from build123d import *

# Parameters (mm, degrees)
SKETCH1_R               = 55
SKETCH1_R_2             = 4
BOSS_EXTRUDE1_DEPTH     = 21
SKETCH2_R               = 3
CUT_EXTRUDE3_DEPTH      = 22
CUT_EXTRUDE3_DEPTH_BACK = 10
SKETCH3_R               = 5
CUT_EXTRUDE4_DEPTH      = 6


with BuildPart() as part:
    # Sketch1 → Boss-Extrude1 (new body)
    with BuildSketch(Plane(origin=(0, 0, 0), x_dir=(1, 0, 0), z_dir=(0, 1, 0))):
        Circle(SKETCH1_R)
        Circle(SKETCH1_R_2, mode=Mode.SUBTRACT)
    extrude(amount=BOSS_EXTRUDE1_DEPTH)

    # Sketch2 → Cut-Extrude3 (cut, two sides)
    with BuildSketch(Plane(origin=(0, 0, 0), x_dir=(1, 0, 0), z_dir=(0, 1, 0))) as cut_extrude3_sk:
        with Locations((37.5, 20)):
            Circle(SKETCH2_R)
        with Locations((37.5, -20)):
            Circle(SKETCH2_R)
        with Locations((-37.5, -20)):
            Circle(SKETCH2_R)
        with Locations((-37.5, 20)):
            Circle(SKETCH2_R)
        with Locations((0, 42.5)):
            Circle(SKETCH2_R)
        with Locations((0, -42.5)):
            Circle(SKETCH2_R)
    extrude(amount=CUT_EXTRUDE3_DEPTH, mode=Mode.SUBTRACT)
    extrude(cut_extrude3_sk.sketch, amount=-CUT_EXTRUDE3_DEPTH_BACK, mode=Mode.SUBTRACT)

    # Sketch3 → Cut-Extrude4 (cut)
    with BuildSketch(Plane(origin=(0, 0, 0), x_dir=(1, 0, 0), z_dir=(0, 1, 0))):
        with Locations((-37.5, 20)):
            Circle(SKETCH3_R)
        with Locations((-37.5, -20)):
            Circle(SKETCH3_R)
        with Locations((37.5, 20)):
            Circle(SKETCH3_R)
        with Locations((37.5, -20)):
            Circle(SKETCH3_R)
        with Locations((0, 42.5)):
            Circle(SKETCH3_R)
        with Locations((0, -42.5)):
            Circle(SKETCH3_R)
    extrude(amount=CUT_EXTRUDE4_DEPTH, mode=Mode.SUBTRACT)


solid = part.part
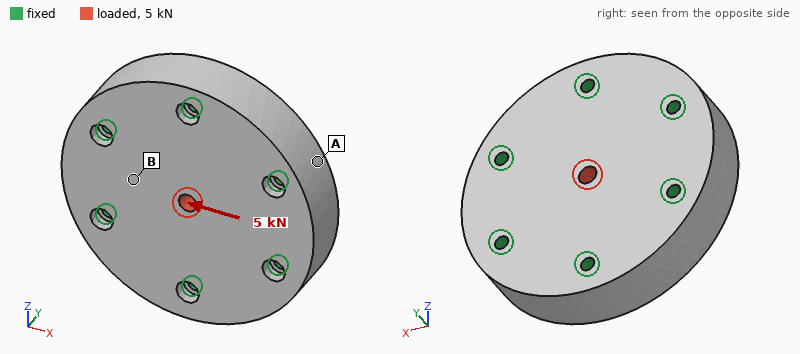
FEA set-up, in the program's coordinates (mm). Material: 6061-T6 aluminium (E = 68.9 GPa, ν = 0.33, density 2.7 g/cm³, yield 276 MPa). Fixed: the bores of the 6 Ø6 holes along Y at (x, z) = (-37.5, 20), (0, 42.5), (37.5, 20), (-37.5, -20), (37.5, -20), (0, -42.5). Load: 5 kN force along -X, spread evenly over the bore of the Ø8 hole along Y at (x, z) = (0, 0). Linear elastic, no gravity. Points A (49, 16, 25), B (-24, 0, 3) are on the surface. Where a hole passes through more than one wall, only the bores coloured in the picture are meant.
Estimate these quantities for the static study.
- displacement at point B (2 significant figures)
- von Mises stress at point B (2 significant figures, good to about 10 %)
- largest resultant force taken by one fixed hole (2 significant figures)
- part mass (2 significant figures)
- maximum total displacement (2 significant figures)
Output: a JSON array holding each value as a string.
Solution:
["1.1 µm", "2.5 MPa", "1.1 kN", "520 g", "2.6 µm"]
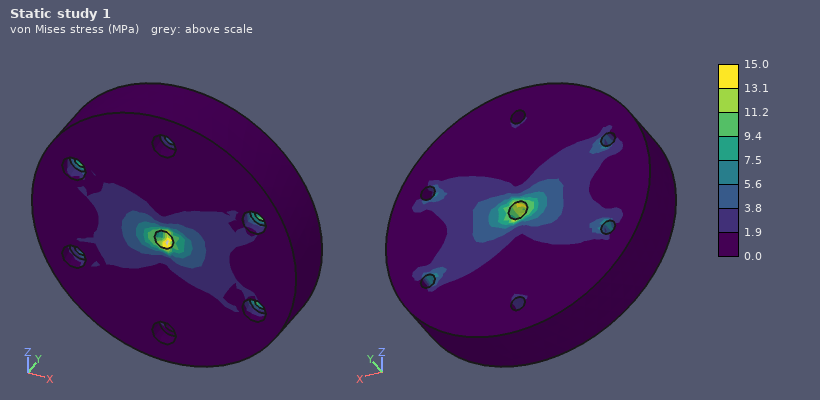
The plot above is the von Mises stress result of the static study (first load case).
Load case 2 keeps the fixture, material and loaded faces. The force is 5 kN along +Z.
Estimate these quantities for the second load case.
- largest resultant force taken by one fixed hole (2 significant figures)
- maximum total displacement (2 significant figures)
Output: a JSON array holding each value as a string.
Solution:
["1.3 kN", "2.6 µm"]
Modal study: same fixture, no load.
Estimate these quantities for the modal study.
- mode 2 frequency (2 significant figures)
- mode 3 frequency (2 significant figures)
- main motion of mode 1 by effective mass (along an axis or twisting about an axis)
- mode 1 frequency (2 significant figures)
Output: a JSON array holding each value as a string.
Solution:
["20 kHz", "20 kHz", "along Y", "14 kHz"]
